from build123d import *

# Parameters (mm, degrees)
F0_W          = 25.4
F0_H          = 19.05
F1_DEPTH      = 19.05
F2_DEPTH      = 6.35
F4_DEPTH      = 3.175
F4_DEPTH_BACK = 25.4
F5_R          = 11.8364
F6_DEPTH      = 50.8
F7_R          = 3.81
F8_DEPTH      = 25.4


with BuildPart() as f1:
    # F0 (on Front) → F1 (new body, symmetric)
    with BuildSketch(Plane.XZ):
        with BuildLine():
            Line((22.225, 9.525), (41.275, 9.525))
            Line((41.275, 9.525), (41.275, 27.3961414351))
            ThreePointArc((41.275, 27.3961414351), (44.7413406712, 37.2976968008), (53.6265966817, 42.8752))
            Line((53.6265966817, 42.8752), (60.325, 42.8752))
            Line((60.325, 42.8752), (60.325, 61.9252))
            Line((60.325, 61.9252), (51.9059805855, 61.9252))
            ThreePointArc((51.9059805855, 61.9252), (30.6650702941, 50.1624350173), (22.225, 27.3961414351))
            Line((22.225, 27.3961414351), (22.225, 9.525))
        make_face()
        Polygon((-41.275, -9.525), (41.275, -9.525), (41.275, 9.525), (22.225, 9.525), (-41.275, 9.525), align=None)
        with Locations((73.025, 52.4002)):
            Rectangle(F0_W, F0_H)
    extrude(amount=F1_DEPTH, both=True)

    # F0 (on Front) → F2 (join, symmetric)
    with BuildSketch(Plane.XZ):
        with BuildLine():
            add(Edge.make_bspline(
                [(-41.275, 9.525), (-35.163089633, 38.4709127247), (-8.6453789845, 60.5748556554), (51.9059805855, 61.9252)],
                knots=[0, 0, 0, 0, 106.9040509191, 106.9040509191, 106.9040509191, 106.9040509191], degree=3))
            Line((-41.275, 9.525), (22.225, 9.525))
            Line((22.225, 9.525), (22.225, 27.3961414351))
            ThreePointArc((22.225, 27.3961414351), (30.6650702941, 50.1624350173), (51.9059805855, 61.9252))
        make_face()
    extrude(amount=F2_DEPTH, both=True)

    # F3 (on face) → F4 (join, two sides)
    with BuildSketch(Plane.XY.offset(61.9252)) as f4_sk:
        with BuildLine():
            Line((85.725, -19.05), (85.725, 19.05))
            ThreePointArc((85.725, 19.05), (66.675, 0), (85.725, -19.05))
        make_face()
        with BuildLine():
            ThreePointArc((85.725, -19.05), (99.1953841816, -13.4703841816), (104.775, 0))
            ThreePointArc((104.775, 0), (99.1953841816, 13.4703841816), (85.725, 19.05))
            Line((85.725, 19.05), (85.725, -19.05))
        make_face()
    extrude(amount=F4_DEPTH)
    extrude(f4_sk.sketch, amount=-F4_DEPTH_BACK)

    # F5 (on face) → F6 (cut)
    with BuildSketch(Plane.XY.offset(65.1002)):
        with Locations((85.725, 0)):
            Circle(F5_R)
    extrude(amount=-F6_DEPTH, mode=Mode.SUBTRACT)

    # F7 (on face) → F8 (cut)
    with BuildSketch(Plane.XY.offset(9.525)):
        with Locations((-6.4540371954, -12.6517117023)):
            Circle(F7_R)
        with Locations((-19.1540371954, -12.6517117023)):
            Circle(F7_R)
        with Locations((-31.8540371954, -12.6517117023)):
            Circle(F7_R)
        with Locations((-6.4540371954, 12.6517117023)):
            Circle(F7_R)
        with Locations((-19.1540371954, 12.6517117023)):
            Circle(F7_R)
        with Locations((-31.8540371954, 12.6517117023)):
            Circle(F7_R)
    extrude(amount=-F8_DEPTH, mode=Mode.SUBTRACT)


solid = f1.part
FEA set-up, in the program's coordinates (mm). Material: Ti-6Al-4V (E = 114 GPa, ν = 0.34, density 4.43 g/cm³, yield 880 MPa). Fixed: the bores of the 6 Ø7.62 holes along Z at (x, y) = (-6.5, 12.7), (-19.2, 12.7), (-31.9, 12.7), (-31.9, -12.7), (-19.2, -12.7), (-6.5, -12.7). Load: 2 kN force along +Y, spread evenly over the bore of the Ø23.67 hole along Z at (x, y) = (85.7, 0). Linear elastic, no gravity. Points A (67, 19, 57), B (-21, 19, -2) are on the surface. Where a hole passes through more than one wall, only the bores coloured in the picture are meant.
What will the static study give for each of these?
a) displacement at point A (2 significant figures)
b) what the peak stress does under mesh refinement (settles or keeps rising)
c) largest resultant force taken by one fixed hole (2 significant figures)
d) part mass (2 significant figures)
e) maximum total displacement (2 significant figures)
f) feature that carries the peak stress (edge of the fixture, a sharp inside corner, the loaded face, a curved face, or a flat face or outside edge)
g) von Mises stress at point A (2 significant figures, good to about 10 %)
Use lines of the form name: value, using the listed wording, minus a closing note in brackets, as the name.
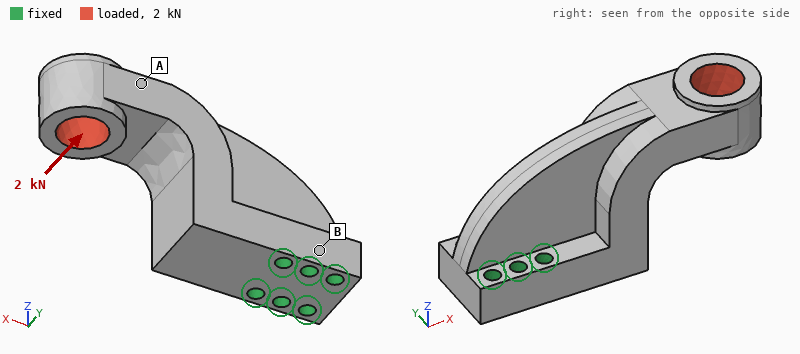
displacement at point A: 0.12 mm
what the peak stress does under mesh refinement: keeps rising
largest resultant force taken by one fixed hole: 6.7 kN
part mass: 700 g
maximum total displacement: 0.19 mm
feature that carries the peak stress: edge of the fixture
von Mises stress at point A: 10 MPa
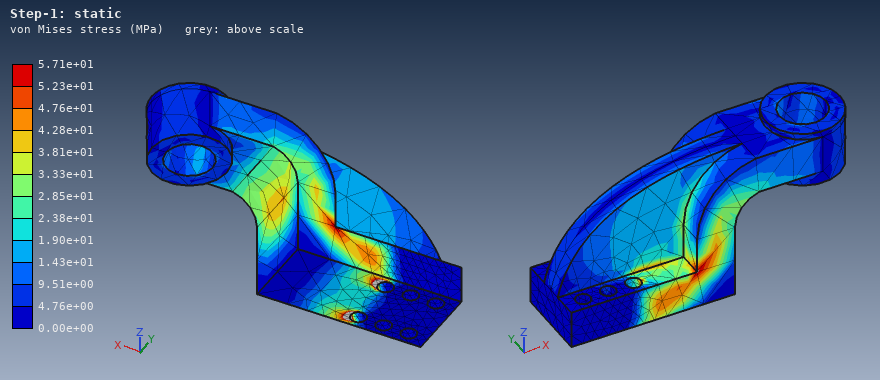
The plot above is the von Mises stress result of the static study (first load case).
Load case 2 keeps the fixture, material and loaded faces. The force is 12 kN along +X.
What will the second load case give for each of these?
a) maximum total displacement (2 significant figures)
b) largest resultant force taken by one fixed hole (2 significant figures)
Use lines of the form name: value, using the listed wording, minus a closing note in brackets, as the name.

maximum total displacement: 0.17 mm
largest resultant force taken by one fixed hole: 6.8 kN
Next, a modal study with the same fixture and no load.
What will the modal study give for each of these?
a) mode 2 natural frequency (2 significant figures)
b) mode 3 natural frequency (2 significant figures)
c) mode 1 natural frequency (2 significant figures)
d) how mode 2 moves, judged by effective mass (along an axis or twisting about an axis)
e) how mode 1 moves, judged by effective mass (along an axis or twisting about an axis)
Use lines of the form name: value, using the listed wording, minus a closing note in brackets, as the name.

mode 2 natural frequency: 2100 Hz
mode 3 natural frequency: 3900 Hz
mode 1 natural frequency: 1500 Hz
how mode 2 moves, judged by effective mass: along Z
how mode 1 moves, judged by effective mass: along Y
